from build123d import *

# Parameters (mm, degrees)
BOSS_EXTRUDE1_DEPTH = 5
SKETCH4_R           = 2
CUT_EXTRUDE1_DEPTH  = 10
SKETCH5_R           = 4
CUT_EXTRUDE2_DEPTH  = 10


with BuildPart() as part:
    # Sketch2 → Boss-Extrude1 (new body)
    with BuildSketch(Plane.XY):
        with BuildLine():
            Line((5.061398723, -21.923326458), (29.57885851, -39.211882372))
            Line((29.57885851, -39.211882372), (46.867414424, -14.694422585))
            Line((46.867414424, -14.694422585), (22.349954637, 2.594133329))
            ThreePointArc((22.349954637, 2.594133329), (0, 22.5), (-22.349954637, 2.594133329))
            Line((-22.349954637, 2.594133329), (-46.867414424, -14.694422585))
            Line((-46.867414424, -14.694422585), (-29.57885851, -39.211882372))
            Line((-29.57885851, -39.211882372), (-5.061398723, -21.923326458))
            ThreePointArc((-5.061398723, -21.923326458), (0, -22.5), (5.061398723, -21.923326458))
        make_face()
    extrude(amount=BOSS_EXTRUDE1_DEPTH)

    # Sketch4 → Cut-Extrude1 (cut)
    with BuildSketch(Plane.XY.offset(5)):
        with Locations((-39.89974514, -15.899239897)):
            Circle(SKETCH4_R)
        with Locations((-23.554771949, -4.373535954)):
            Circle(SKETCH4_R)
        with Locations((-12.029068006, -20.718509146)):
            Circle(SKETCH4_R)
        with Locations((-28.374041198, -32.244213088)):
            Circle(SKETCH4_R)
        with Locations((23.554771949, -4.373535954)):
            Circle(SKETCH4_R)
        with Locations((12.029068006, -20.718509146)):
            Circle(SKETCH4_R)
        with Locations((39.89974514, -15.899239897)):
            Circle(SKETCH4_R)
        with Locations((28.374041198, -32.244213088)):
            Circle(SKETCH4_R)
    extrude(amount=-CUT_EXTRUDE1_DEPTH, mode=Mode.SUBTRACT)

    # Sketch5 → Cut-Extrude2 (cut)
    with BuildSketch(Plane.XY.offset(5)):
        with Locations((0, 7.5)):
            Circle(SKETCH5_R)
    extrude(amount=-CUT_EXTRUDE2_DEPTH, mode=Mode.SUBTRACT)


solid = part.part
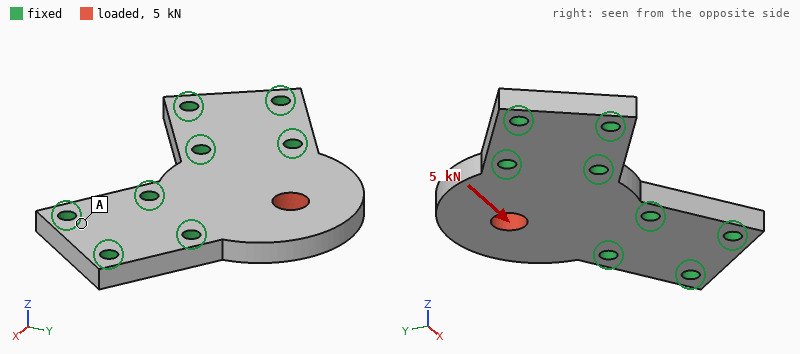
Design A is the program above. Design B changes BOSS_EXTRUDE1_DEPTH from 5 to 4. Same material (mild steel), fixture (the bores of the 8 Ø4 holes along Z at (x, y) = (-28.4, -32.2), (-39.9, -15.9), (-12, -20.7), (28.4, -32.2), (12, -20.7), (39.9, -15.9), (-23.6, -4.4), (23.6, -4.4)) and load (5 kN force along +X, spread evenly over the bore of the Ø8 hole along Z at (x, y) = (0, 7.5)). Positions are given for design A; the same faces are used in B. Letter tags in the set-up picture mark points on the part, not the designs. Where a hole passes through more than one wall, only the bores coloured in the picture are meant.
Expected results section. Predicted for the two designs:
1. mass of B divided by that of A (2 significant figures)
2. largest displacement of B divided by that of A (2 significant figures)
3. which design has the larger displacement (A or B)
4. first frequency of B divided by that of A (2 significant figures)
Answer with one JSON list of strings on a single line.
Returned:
["0.80", "1.3", "B", "0.82"]
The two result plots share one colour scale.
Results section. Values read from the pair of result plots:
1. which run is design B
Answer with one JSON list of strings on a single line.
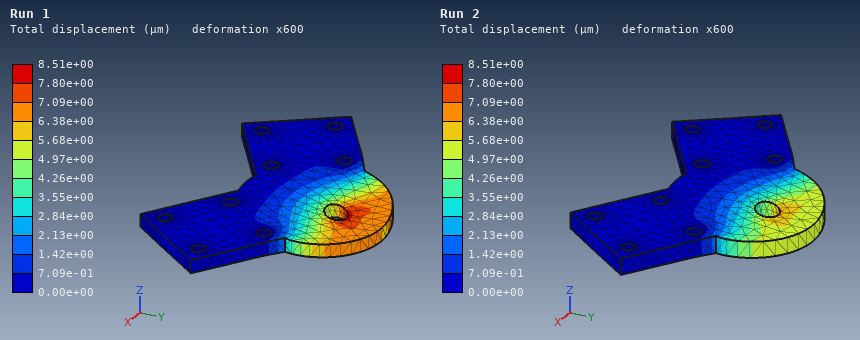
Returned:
["Run 1"]
